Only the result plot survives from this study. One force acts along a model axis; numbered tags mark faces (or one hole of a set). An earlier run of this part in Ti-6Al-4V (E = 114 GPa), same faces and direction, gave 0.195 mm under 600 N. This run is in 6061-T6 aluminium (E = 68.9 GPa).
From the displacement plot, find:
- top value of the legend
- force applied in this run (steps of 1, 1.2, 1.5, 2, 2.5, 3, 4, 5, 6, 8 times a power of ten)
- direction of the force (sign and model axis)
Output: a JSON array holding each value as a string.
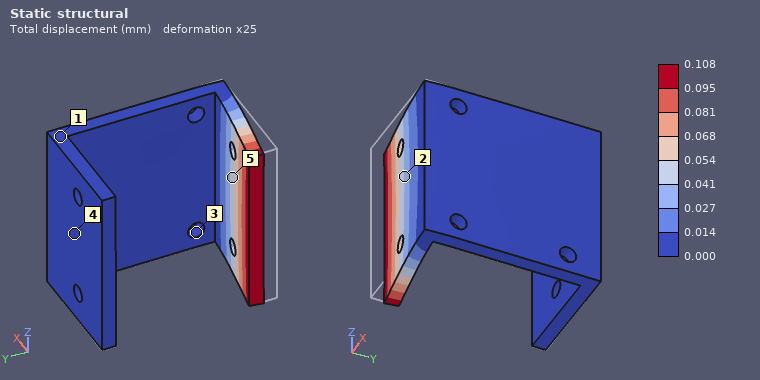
["0.108 mm", "200 N", "+Y"]
